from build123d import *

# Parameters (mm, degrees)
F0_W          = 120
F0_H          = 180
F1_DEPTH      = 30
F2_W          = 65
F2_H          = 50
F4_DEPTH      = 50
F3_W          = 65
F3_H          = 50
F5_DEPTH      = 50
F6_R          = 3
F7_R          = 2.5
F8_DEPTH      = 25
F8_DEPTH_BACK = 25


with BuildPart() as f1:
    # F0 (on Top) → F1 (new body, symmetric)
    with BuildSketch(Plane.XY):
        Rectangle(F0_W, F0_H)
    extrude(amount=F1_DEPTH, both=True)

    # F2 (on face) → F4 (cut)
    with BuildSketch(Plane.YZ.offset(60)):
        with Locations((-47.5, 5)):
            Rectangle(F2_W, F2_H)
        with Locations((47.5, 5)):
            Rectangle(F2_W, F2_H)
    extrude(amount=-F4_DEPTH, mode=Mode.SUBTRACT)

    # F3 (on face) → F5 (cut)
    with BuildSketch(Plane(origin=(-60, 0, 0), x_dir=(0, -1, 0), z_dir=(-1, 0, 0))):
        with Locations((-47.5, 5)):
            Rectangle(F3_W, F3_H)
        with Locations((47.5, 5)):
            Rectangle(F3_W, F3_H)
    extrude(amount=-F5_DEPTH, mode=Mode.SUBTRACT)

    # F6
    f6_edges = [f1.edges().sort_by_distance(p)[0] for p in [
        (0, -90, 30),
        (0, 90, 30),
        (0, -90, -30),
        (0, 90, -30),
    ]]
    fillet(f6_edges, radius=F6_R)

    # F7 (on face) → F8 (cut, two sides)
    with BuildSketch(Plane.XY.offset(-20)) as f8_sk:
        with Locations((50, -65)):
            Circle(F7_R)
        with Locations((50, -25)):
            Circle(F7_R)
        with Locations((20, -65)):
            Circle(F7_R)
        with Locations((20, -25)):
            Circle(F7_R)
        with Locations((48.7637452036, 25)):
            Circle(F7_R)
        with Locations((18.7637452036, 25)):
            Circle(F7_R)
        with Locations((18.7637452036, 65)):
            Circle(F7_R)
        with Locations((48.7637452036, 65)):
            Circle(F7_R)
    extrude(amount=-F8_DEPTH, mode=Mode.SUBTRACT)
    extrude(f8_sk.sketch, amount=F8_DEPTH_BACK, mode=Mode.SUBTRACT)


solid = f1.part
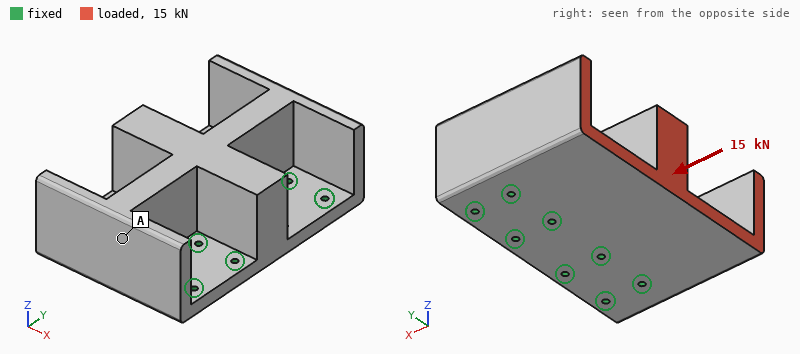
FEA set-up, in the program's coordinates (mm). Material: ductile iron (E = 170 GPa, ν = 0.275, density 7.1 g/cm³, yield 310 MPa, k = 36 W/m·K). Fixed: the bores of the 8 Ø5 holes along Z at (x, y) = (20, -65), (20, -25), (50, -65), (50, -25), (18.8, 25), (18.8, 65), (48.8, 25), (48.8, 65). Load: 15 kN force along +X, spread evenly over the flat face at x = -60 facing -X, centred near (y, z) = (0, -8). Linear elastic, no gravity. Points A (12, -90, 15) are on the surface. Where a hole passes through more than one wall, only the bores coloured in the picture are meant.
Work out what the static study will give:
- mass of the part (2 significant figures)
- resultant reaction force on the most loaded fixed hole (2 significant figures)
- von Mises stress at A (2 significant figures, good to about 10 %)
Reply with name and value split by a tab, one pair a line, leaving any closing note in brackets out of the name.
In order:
mass of the part	4.6 kg
resultant reaction force on the most loaded fixed hole	3.2 kN
von Mises stress at A	6.1 MPa
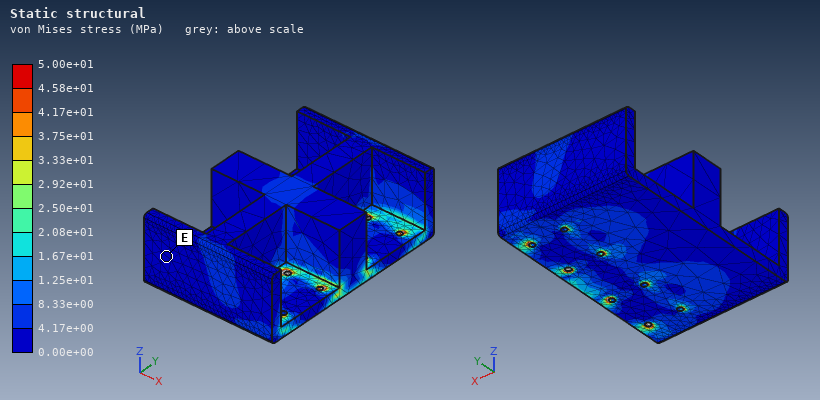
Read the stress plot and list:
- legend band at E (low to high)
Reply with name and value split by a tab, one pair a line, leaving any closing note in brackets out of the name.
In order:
legend band at E	0.00e+00 to 4.17e+00 MPa
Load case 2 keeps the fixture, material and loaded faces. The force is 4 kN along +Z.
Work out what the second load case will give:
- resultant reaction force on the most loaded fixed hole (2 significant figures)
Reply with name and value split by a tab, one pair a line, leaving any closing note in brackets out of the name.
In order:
resultant reaction force on the most loaded fixed hole	3.5 kN
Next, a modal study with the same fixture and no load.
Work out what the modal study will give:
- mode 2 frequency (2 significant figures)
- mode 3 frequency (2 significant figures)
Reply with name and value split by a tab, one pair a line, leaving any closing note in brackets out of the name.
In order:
mode 2 frequency	2200 Hz
mode 3 frequency	3700 Hz
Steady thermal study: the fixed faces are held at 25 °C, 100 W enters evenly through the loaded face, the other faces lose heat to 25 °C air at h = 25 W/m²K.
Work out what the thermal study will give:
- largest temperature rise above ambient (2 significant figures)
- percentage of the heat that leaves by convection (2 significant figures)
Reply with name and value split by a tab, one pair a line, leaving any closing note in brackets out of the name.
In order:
largest temperature rise above ambient	51 K
percentage of the heat that leaves by convection	44 %
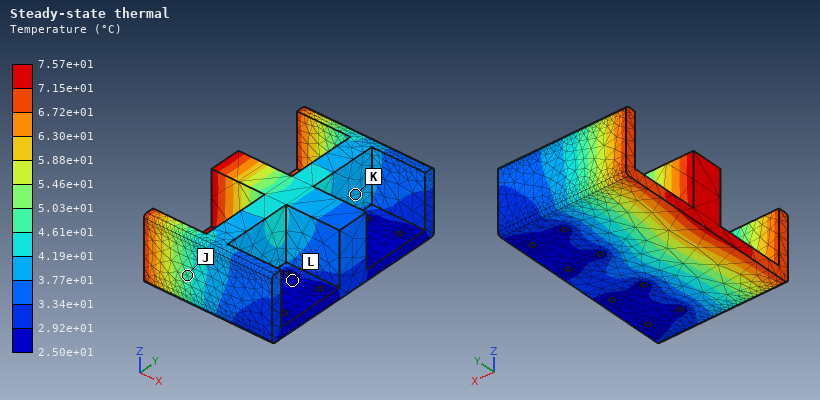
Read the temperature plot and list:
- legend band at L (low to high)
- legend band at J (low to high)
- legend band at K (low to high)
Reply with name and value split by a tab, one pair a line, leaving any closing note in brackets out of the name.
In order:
legend band at L	2.50e+01 to 2.92e+01 °C
legend band at J	4.61e+01 to 5.03e+01 °C
legend band at K	3.77e+01 to 4.19e+01 °C
